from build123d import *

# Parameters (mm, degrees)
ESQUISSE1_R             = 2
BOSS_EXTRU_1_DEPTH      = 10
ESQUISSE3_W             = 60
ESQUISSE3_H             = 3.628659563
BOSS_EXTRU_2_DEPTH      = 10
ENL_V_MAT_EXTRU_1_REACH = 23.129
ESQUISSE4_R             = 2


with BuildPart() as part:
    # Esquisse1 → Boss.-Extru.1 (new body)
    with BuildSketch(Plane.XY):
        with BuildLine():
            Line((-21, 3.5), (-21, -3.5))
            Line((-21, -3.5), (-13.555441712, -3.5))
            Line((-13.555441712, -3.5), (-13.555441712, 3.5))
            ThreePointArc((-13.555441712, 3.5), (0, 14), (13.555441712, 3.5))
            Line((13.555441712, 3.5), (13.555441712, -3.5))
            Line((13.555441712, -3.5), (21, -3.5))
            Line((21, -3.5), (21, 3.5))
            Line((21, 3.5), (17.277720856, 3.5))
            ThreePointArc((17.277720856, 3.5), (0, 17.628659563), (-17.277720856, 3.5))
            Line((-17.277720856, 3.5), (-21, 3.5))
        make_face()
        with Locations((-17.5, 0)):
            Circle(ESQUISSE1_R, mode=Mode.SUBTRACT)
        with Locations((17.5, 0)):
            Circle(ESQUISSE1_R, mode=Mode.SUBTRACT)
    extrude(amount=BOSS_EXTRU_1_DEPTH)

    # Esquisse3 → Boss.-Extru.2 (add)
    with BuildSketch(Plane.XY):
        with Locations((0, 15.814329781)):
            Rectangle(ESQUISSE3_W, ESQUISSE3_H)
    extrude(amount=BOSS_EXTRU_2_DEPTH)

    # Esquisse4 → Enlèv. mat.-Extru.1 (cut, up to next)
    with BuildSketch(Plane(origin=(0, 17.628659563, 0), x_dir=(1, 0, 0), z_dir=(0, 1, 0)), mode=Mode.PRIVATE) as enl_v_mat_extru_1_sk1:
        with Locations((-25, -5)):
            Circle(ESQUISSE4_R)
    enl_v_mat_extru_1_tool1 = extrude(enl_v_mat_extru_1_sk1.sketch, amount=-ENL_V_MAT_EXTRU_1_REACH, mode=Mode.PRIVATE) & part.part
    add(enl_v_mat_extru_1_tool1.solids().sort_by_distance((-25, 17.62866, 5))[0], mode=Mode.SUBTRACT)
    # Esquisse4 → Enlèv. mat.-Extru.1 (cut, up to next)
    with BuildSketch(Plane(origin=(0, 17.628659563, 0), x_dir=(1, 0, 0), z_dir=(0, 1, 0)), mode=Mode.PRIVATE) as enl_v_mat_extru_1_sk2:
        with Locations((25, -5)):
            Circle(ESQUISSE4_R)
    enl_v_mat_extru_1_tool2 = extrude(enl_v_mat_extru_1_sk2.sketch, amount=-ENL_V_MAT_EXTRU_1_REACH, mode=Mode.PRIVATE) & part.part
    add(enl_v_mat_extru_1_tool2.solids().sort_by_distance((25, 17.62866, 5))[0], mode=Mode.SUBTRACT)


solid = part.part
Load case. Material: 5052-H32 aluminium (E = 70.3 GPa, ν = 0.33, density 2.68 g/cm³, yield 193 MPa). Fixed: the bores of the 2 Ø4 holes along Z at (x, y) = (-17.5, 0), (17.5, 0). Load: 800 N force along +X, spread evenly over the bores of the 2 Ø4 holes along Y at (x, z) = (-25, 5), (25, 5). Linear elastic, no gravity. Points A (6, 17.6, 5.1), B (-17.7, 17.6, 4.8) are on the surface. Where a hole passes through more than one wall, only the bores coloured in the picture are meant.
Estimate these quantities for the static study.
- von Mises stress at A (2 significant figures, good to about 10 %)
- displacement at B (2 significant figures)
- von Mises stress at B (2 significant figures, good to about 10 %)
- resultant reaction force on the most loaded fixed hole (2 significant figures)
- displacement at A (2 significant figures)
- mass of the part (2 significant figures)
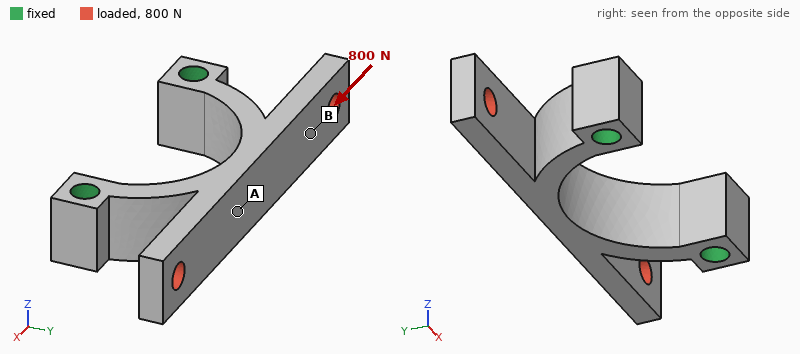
31 MPa
20 µm
11 MPa
460 N
18 µm
10 g
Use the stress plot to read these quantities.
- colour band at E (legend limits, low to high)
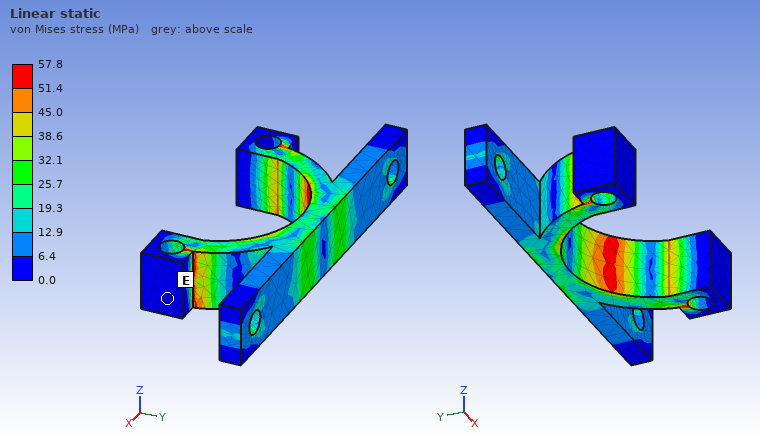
0.0 to 6.4 MPa
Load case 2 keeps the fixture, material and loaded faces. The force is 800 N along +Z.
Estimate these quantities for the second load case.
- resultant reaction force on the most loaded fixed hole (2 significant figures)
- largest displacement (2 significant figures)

400 N
0.13 mm
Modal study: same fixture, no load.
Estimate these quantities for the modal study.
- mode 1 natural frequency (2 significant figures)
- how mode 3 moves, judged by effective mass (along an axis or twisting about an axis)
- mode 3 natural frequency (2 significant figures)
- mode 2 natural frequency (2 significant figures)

6100 Hz
twisting about Y
7900 Hz
6300 Hz
